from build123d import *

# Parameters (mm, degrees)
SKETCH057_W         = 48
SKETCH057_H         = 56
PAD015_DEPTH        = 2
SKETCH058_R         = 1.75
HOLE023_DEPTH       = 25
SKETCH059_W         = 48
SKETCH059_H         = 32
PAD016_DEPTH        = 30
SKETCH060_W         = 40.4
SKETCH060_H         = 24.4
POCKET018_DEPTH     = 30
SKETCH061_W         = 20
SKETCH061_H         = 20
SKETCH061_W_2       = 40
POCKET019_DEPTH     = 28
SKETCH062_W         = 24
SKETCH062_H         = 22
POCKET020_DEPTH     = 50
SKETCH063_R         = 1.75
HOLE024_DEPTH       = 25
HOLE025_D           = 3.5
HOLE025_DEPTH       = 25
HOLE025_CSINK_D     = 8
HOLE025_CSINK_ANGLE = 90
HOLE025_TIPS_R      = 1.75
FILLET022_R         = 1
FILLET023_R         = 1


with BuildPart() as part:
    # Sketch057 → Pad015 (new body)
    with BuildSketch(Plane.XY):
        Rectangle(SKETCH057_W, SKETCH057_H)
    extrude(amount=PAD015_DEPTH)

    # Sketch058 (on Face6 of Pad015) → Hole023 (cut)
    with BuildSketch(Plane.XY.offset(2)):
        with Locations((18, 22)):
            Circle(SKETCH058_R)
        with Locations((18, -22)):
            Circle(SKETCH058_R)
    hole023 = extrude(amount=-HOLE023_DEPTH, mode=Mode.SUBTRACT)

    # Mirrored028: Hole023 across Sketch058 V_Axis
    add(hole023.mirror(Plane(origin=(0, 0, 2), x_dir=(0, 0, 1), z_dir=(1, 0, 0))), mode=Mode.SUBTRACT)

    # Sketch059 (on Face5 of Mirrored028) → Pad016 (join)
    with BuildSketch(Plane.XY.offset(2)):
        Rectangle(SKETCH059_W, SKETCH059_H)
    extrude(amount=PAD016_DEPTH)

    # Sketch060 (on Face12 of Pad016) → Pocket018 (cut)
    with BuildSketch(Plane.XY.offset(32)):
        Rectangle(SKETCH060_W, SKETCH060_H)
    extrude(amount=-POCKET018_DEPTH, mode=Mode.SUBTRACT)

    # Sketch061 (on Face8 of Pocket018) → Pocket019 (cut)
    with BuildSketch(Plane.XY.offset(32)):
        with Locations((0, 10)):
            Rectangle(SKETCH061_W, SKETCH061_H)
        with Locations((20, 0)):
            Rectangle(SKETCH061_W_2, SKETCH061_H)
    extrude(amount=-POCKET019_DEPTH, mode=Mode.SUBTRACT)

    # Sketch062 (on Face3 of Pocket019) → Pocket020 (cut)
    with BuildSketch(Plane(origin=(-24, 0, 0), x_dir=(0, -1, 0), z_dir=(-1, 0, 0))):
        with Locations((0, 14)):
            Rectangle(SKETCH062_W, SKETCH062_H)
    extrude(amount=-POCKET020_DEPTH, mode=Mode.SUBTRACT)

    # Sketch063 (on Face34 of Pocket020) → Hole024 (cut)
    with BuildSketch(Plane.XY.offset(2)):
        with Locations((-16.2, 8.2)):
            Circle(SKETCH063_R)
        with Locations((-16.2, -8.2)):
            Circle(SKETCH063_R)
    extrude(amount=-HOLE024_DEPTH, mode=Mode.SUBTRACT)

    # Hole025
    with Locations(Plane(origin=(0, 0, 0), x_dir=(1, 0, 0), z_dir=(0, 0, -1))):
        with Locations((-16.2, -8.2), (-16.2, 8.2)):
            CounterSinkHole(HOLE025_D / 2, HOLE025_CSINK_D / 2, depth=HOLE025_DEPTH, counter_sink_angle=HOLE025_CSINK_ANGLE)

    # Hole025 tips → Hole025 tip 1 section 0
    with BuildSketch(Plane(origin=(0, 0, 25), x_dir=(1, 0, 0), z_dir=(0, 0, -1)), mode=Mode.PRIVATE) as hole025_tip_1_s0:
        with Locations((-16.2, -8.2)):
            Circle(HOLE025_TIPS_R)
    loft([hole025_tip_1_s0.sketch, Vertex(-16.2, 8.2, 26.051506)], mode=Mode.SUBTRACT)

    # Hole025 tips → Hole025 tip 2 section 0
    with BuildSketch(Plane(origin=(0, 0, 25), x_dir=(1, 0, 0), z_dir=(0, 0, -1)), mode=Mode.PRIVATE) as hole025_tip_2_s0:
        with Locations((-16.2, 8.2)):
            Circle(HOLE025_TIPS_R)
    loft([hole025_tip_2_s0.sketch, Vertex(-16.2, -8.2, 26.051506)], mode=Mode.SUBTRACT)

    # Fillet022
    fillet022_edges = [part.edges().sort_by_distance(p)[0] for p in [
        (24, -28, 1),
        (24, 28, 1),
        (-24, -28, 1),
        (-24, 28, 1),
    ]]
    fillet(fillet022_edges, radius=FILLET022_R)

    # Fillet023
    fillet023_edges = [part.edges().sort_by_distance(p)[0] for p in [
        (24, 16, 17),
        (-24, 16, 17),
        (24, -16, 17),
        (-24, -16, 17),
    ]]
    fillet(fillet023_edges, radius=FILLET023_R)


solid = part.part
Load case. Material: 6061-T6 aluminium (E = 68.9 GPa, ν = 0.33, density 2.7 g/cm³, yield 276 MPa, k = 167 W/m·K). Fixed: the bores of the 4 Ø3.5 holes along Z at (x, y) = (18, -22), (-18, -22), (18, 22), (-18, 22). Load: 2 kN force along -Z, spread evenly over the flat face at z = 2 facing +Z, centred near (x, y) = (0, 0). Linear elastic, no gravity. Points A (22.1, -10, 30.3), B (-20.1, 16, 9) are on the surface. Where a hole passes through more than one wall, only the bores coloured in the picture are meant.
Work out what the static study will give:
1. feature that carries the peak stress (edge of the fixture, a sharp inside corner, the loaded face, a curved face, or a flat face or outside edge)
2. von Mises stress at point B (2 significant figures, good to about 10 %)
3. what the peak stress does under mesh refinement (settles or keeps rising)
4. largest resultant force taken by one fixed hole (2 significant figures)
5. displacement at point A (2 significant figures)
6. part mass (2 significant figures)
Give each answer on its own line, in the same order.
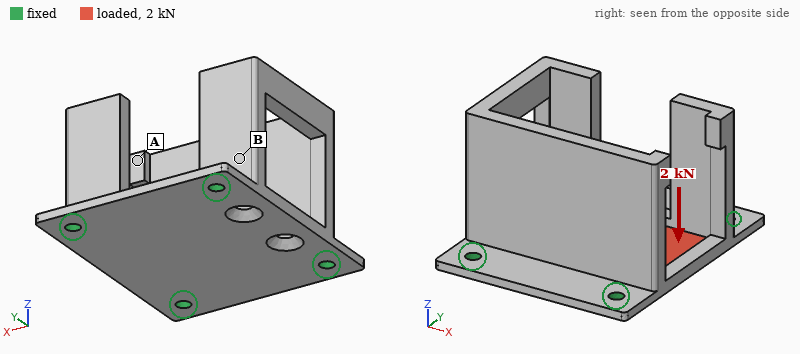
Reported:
edge of the fixture
84 MPa
keeps rising
650 N
0.27 mm
40 g
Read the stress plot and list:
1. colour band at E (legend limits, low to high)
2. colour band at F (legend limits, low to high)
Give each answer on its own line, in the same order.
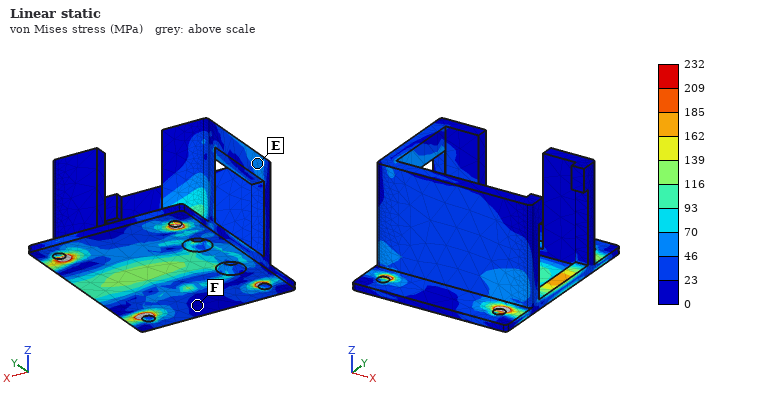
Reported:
46 to 70 MPa
0 to 23 MPa
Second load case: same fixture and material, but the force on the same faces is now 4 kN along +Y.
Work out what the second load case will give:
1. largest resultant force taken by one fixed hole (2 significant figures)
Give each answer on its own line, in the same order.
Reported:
1.1 kN
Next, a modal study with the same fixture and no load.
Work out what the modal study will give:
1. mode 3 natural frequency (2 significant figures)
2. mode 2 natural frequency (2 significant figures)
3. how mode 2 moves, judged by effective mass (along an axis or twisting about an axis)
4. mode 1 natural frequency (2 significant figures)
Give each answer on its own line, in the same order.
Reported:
3300 Hz
2600 Hz
along Y
2000 Hz
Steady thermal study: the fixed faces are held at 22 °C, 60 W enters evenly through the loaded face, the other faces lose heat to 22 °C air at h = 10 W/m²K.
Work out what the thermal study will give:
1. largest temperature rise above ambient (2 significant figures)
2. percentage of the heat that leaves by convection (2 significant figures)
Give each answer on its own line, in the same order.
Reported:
39 K
3.5 %
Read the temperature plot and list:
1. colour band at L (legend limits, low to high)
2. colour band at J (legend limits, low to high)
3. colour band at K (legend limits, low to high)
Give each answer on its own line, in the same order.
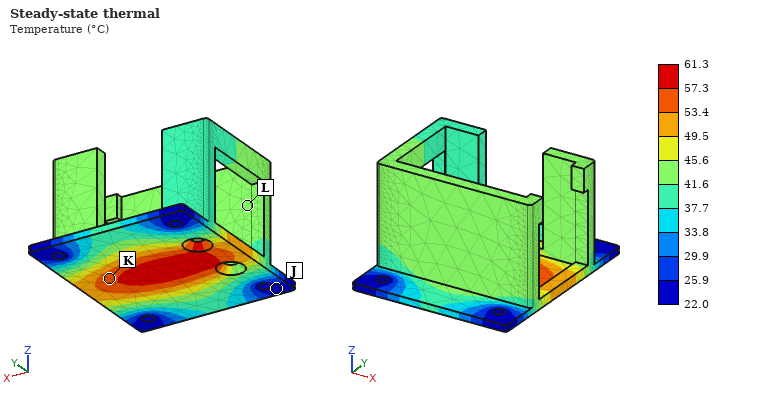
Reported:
41.6 to 45.6 °C
22.0 to 25.9 °C
53.4 to 57.3 °C
